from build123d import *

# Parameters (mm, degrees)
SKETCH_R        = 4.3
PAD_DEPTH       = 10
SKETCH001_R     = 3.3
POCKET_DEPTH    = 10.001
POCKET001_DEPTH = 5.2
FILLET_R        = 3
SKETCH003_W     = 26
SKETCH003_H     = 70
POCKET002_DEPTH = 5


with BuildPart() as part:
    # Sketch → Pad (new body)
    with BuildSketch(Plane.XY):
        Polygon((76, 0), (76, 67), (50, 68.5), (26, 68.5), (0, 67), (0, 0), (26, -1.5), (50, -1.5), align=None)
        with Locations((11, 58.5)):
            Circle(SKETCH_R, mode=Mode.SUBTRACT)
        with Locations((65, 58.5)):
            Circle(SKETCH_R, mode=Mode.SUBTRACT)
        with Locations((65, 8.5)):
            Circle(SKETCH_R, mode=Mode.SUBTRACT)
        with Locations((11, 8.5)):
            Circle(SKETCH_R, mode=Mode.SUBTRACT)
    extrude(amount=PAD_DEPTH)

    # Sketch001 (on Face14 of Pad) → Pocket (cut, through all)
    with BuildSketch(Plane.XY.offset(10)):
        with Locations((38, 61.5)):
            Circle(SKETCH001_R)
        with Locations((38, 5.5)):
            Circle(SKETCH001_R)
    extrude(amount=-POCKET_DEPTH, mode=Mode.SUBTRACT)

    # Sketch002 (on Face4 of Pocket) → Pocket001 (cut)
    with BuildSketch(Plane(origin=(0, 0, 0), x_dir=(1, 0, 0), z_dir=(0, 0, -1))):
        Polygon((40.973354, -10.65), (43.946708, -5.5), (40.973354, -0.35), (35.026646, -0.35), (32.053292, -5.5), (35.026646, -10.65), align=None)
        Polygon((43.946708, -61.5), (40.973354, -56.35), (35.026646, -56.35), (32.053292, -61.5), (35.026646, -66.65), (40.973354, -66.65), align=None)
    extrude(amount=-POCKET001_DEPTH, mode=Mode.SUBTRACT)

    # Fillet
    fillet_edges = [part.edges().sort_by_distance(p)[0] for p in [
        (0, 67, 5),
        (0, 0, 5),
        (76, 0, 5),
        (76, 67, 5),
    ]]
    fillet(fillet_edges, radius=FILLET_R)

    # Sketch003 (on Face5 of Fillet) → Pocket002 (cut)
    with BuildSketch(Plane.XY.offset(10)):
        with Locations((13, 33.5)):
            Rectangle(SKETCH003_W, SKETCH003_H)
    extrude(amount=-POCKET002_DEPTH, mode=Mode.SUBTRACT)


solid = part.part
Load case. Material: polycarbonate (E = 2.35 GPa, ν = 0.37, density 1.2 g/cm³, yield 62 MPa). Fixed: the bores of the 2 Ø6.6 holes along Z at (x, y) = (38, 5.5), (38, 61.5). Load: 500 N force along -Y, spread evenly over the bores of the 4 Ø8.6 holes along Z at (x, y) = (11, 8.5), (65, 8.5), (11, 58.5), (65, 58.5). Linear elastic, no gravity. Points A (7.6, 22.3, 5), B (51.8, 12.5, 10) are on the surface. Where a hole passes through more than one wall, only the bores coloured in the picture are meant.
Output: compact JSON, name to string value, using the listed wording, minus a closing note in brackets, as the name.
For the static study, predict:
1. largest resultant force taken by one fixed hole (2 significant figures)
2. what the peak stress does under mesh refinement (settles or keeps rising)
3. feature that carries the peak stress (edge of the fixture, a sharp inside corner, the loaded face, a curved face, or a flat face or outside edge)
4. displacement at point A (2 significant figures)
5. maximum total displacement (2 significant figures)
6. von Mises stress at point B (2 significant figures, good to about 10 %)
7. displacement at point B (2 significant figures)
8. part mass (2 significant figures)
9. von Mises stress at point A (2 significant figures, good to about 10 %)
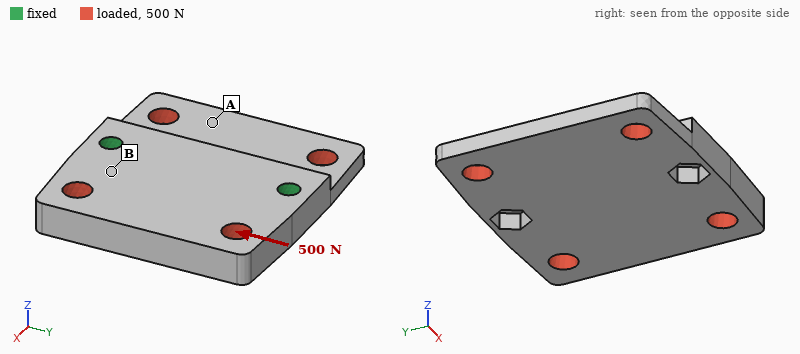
{"largest resultant force taken by one fixed hole": "260 N", "what the peak stress does under mesh refinement": "keeps rising", "feature that carries the peak stress": "edge of the fixture", "displacement at point A": "24 µm", "maximum total displacement": "39 µm", "von Mises stress at point B": "1.5 MPa", "displacement at point B": "18 µm", "part mass": "49 g", "von Mises stress at point A": "0.60 MPa"}
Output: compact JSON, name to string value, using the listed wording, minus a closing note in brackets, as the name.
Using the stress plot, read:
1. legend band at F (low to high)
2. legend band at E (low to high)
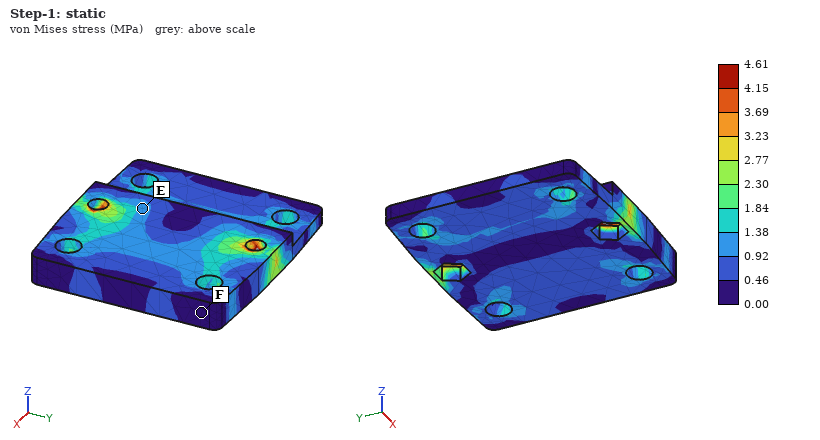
{"legend band at F": "0.00 to 0.46 MPa", "legend band at E": "0.92 to 1.38 MPa"}
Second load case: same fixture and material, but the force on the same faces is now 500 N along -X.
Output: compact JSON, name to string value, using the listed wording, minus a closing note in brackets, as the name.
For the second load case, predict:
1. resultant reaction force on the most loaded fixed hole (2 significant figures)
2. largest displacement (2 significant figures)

{"resultant reaction force on the most loaded fixed hole": "250 N", "largest displacement": "0.13 mm"}
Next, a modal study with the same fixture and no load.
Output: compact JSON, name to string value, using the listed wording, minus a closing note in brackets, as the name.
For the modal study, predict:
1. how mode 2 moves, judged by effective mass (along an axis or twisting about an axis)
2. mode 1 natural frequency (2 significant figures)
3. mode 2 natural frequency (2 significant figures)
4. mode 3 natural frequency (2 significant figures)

{"how mode 2 moves, judged by effective mass": "along Z", "mode 1 natural frequency": "740 Hz", "mode 2 natural frequency": "1300 Hz", "mode 3 natural frequency": "1700 Hz"}
